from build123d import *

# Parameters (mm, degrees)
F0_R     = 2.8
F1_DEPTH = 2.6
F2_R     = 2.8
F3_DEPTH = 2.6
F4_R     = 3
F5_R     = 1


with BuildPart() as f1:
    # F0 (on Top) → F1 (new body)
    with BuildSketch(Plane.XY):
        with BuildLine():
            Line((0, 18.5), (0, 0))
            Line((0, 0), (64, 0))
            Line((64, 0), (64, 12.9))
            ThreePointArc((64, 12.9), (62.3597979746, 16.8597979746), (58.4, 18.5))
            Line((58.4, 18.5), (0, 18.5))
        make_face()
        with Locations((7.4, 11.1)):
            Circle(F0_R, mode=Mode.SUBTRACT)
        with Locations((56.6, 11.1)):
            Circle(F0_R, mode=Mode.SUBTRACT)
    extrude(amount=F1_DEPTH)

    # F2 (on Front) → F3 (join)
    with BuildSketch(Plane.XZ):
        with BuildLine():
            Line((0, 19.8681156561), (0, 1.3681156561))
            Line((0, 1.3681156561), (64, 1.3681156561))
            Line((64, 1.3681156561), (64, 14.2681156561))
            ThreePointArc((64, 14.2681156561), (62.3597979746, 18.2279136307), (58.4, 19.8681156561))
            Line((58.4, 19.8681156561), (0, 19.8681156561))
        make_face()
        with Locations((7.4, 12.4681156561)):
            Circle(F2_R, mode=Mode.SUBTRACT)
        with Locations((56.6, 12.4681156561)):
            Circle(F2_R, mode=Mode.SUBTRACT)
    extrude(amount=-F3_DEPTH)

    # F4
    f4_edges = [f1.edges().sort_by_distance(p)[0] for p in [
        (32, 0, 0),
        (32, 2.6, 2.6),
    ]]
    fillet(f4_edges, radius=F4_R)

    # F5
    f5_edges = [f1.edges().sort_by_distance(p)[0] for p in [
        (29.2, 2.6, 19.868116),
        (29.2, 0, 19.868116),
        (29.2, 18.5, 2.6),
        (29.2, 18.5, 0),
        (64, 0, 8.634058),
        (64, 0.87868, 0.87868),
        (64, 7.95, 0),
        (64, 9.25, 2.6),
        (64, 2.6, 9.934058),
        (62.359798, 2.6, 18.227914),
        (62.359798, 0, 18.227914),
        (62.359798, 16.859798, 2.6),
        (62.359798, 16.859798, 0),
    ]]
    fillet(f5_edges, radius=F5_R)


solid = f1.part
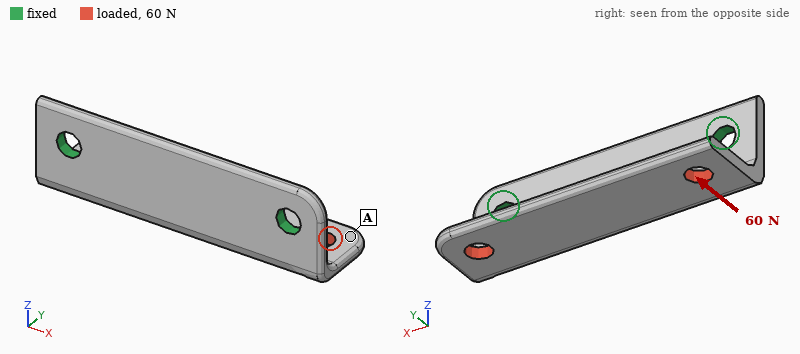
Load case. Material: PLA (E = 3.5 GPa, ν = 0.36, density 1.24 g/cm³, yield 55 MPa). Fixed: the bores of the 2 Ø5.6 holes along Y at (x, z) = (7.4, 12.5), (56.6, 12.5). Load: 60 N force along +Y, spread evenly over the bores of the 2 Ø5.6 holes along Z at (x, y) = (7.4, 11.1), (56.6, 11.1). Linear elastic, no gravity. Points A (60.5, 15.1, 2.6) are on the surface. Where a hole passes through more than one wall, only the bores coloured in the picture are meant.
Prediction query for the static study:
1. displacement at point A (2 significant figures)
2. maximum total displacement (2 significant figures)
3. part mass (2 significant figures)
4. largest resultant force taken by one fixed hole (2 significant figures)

0.18 mm
0.22 mm
6.9 g
30 N
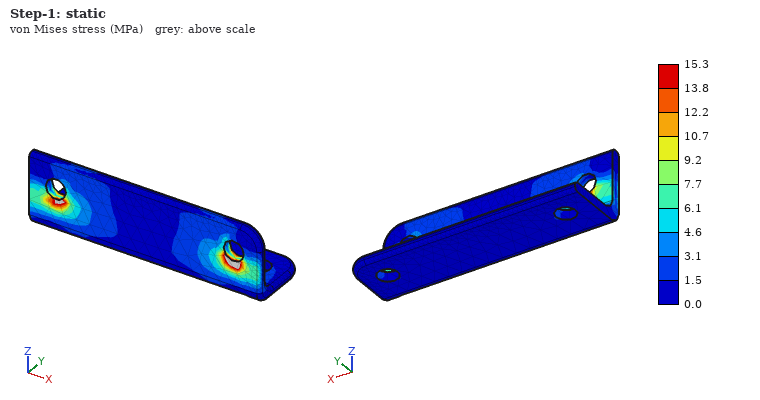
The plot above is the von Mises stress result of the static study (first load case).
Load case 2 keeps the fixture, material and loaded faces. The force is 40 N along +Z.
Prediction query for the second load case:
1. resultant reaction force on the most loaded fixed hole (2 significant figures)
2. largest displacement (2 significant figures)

20 N
0.30 mm
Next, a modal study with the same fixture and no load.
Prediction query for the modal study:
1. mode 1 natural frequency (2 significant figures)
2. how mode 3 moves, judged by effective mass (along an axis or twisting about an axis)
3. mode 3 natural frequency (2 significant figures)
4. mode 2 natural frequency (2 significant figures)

1200 Hz
along Y
2600 Hz
2000 Hz
